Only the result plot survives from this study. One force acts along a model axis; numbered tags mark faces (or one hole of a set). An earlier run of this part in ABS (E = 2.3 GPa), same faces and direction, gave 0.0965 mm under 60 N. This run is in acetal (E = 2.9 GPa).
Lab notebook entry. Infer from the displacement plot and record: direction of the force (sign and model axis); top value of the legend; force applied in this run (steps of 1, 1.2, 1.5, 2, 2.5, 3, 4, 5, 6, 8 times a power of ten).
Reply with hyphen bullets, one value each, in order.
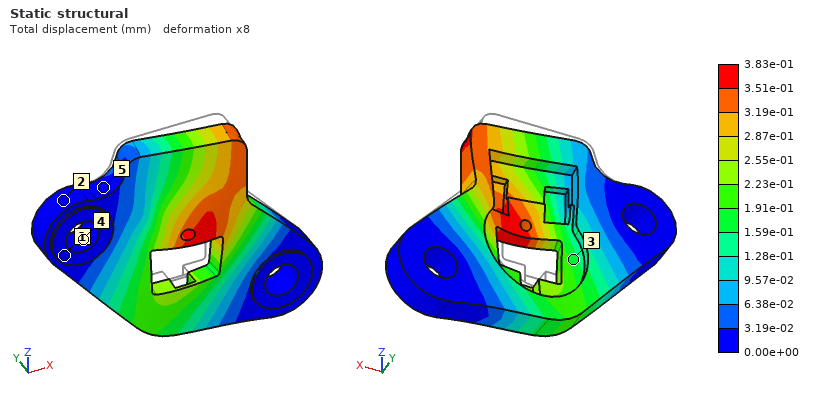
- -Y
- 3.83e-01 mm
- 300 N
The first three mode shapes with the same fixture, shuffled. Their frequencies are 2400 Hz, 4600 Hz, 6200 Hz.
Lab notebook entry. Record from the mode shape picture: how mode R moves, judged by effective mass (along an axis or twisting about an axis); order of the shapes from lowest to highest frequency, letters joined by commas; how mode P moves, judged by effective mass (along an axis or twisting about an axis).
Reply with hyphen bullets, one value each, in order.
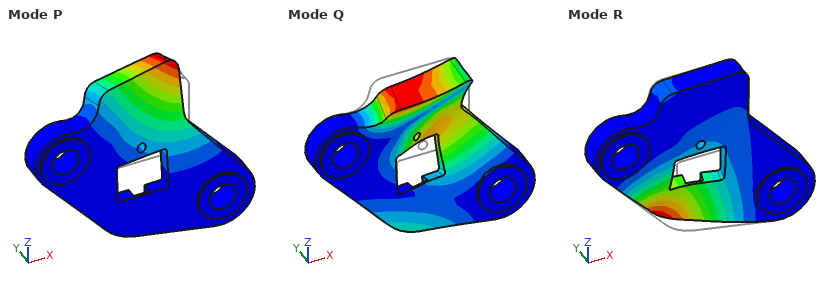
- along Y
- P, R, Q
- along Y
